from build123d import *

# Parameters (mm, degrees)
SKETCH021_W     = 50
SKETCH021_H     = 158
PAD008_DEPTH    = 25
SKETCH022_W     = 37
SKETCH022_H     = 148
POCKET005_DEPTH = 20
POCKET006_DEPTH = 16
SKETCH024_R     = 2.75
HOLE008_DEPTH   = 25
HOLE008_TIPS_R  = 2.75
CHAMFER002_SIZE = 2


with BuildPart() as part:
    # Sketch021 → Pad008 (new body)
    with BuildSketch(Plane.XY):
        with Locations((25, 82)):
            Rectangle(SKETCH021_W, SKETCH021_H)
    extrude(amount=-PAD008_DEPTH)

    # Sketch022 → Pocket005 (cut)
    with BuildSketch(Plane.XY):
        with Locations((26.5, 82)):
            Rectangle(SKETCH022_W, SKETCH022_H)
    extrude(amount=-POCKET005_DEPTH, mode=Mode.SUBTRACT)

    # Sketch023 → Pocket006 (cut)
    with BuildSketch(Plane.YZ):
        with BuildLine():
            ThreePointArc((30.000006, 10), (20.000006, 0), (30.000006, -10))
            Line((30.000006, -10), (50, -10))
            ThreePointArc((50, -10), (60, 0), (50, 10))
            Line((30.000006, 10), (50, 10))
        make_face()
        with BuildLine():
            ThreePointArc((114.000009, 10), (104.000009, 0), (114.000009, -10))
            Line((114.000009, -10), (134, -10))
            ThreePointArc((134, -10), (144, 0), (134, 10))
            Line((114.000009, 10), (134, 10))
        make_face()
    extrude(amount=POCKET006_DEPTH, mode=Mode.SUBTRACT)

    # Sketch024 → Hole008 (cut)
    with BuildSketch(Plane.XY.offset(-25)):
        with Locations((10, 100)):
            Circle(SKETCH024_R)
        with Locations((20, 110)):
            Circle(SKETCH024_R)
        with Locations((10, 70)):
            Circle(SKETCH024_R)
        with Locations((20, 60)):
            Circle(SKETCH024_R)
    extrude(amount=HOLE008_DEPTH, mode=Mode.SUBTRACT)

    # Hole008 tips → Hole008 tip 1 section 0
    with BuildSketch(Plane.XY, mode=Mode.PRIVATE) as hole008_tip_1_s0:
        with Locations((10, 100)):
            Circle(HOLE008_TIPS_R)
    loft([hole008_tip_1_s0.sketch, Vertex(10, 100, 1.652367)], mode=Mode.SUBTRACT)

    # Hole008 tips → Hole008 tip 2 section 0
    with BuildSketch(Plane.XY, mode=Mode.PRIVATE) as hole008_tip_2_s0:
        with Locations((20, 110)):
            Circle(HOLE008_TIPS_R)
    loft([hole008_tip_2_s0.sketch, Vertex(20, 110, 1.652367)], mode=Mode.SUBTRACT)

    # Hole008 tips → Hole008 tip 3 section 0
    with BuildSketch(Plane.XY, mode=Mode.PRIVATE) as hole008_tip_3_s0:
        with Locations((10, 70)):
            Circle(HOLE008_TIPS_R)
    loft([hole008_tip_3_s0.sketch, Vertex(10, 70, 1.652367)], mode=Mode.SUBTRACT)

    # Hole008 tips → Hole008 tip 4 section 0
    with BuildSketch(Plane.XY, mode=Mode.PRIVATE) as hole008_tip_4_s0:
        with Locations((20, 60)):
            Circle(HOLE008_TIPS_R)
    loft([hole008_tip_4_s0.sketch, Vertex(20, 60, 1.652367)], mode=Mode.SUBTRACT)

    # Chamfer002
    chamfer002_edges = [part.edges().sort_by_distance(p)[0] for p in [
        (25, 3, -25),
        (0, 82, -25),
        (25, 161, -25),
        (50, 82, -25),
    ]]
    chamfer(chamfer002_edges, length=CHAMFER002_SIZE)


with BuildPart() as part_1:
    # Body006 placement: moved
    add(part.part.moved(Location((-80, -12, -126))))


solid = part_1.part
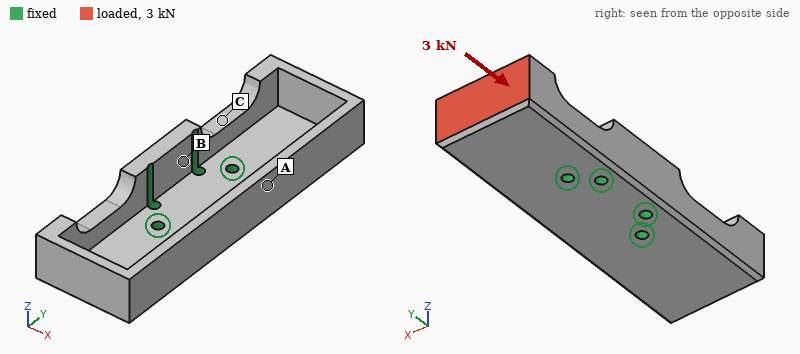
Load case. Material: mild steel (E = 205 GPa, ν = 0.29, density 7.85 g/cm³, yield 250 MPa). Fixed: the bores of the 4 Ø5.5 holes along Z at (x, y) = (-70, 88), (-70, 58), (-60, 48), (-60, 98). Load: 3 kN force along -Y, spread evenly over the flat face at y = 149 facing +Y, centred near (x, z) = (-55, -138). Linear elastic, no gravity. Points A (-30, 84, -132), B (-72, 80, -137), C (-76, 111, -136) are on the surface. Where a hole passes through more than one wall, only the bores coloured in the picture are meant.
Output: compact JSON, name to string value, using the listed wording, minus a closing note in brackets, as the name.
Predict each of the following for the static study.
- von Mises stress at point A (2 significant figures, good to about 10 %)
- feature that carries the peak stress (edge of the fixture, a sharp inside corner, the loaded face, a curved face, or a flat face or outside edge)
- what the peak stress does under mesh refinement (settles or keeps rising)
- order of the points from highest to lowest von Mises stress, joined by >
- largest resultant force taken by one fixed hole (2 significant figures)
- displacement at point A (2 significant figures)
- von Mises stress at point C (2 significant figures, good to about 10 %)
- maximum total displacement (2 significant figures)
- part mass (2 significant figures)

{"von Mises stress at point A": "13 MPa", "feature that carries the peak stress": "edge of the fixture", "what the peak stress does under mesh refinement": "keeps rising", "order of the points from highest to lowest von Mises stress, joined by >": "C > A > B", "largest resultant force taken by one fixed hole": "1.2 kN", "displacement at point A": "7.5 µm", "von Mises stress at point C": "41 MPa", "maximum total displacement": "41 µm", "part mass": "640 g"}
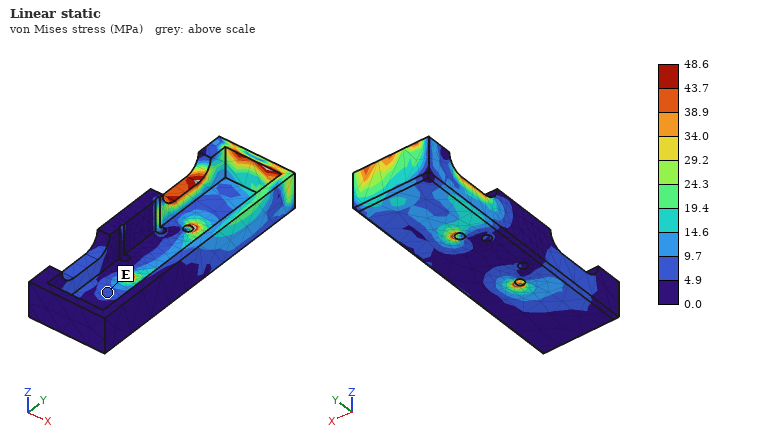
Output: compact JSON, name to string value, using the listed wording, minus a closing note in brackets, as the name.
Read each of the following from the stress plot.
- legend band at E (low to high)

{"legend band at E": "4.9 to 9.7 MPa"}
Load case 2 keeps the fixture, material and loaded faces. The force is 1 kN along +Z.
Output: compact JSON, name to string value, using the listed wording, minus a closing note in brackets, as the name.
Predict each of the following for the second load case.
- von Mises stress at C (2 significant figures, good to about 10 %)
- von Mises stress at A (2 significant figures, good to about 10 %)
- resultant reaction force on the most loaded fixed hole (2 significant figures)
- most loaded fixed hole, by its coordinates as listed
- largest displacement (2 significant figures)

{"von Mises stress at C": "57 MPa", "von Mises stress at A": "20 MPa", "resultant reaction force on the most loaded fixed hole": "1.9 kN", "most loaded fixed hole, by its coordinates as listed": "(-60, 98)", "largest displacement": "83 µm"}
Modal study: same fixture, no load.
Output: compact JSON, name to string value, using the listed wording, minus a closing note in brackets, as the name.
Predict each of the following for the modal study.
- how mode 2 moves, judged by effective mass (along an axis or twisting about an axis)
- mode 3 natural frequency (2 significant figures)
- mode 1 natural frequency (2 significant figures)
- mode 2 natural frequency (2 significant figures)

{"how mode 2 moves, judged by effective mass": "along Z", "mode 3 natural frequency": "2600 Hz", "mode 1 natural frequency": "1500 Hz", "mode 2 natural frequency": "1800 Hz"}
